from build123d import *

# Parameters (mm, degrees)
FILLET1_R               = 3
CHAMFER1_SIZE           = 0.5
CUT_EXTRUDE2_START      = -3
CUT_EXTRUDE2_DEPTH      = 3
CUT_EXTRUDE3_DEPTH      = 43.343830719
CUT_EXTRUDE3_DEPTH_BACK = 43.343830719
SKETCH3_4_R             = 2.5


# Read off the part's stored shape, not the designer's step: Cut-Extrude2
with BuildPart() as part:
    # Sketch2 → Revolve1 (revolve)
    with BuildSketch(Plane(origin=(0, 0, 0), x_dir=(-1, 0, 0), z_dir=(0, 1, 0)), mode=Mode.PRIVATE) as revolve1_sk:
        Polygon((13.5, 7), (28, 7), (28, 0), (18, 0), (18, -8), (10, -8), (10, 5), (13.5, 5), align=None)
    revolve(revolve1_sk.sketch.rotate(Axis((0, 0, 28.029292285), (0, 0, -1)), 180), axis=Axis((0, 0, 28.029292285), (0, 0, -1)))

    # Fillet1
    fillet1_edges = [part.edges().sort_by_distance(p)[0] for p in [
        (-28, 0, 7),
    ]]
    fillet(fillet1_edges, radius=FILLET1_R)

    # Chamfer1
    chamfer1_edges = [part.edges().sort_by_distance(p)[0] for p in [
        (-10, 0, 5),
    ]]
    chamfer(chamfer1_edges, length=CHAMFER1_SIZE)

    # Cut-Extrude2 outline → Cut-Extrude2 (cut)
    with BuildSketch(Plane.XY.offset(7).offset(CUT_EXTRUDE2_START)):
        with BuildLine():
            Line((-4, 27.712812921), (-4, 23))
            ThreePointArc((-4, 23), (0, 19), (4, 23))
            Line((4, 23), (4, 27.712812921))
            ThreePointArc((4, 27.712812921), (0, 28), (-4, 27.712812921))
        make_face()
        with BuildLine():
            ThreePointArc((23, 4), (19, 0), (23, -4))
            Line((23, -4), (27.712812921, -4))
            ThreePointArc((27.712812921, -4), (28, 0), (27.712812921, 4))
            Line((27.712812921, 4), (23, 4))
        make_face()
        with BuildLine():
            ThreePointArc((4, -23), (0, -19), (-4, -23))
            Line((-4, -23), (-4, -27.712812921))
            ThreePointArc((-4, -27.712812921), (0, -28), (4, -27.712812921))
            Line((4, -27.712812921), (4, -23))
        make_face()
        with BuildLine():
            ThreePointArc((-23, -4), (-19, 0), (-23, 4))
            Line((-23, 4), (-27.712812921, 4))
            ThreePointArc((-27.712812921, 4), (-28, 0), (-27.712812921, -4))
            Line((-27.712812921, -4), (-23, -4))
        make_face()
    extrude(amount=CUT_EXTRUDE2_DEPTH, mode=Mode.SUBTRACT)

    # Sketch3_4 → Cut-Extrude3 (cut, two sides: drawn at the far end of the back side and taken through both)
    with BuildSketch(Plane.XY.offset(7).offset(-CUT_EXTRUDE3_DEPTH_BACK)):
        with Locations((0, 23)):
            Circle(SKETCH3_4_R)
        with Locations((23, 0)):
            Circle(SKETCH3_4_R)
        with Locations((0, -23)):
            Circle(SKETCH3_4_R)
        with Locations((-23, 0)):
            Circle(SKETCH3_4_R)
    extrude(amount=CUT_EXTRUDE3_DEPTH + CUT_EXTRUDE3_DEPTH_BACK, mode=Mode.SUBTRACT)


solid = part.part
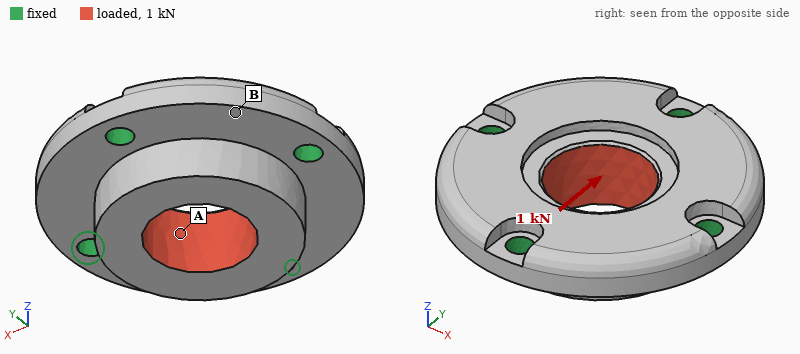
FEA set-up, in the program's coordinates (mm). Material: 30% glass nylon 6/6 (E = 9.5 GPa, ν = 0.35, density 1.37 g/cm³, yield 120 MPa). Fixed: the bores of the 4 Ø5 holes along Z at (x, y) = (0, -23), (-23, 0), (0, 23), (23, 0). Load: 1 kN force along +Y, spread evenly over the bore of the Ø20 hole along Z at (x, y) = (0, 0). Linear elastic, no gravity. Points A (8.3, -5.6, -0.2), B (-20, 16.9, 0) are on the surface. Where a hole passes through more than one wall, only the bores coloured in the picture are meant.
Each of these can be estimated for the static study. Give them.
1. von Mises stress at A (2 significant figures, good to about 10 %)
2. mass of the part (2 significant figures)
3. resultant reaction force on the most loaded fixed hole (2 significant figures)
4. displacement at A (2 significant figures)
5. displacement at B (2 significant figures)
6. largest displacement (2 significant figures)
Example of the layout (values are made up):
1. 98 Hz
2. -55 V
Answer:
1. 2.6 MPa
2. 26 g
3. 290 N
4. 6.4 µm
5. 4.4 µm
6. 9.1 µm
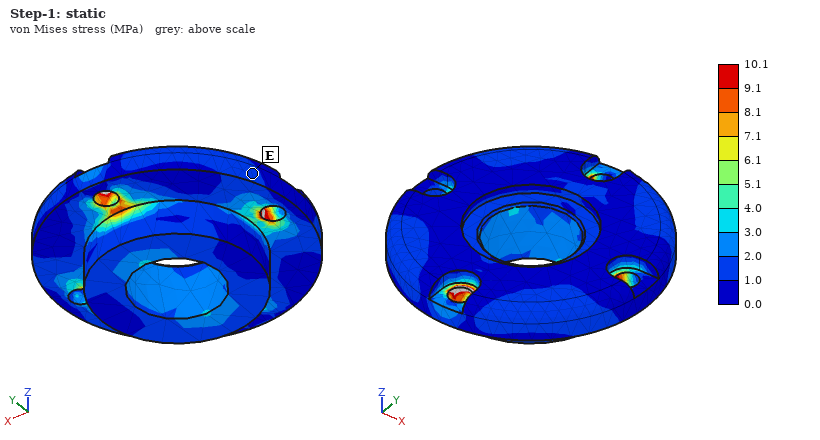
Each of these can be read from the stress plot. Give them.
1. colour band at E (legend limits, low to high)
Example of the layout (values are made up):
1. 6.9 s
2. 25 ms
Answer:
1. 1.0 to 2.0 MPa
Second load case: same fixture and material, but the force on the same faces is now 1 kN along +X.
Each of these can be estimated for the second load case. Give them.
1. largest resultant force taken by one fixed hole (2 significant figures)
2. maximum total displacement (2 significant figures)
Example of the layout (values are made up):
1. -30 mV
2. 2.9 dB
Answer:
1. 290 N
2. 9.2 µm
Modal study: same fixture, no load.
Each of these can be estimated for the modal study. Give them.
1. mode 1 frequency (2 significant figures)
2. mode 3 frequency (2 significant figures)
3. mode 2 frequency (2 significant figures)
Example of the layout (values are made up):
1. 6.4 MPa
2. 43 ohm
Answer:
1. 10 kHz
2. 11 kHz
3. 11 kHz
